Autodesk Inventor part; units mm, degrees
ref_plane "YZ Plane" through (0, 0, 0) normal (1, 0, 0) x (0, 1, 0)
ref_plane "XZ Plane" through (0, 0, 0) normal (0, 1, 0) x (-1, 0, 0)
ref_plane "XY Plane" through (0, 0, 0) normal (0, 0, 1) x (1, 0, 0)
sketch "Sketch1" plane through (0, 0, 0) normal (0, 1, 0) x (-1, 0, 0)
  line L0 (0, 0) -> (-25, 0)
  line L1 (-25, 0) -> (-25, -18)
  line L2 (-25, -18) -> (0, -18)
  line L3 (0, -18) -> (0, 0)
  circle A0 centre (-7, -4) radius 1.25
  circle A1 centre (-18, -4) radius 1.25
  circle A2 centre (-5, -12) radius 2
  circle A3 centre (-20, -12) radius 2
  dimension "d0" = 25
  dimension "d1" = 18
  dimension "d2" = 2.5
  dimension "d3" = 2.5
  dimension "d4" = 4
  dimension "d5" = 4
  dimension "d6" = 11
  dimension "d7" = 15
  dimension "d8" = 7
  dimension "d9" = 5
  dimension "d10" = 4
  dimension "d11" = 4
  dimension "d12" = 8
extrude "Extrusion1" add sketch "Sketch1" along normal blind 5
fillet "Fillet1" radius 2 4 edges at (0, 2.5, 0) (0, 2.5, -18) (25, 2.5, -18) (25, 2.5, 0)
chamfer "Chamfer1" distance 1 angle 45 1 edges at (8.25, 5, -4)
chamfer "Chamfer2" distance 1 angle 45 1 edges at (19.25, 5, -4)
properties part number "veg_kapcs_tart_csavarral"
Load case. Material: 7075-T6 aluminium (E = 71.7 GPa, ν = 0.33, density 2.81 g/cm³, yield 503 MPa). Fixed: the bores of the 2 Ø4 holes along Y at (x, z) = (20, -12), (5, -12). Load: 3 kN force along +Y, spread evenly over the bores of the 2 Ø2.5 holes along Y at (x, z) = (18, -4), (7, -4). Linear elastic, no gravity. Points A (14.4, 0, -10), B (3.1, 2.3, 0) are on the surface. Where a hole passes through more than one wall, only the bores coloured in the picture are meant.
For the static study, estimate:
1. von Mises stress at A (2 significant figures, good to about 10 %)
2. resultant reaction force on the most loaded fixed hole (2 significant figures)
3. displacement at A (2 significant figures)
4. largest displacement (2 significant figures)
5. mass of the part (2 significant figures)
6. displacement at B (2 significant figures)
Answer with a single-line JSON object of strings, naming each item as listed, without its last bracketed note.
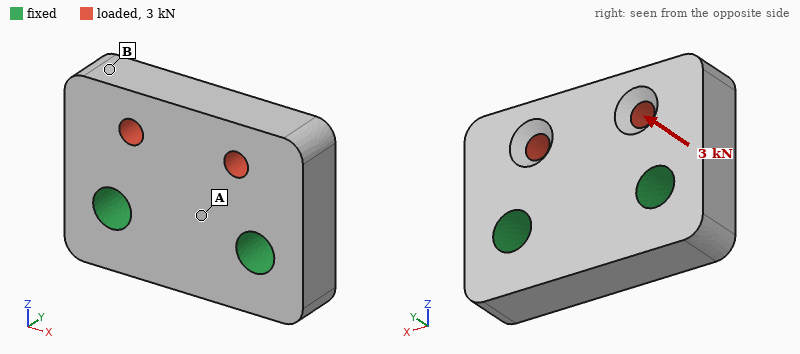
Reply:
{"von Mises stress at A": "88 MPa", "resultant reaction force on the most loaded fixed hole": "1.5 kN", "displacement at A": "11 µm", "largest displacement": "57 µm", "mass of the part": "5.8 g", "displacement at B": "45 µm"}
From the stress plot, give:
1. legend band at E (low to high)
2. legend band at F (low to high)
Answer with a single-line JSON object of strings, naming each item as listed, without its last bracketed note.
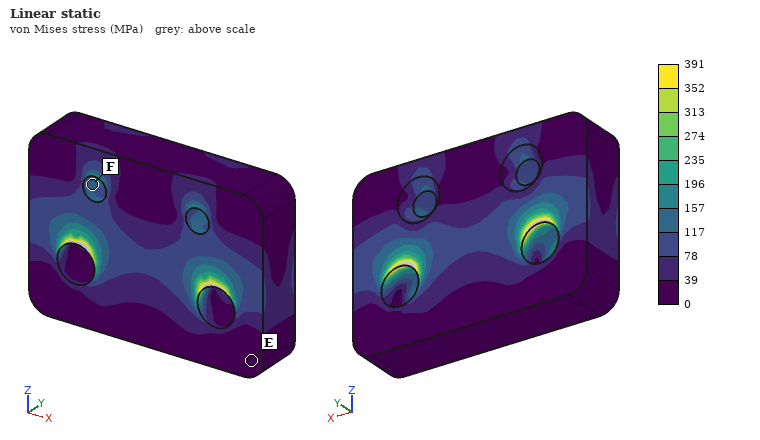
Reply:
{"legend band at E": "0 to 39 MPa", "legend band at F": "117 to 157 MPa"}
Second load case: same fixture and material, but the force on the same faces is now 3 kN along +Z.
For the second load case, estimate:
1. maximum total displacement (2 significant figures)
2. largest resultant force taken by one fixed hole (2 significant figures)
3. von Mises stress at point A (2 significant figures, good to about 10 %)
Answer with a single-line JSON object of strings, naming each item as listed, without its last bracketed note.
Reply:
{"maximum total displacement": "8.2 µm", "largest resultant force taken by one fixed hole": "1.5 kN", "von Mises stress at point A": "21 MPa"}
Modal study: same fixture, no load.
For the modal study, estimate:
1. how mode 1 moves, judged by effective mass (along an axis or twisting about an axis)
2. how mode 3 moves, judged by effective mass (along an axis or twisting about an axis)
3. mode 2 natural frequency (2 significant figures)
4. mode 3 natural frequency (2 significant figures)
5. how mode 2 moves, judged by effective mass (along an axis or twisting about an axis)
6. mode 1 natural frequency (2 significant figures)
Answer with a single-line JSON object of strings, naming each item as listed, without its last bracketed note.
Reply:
{"how mode 1 moves, judged by effective mass": "along Y", "how mode 3 moves, judged by effective mass": "along X", "mode 2 natural frequency": "38 kHz", "mode 3 natural frequency": "54 kHz", "how mode 2 moves, judged by effective mass": "twisting about Z", "mode 1 natural frequency": "28 kHz"}
